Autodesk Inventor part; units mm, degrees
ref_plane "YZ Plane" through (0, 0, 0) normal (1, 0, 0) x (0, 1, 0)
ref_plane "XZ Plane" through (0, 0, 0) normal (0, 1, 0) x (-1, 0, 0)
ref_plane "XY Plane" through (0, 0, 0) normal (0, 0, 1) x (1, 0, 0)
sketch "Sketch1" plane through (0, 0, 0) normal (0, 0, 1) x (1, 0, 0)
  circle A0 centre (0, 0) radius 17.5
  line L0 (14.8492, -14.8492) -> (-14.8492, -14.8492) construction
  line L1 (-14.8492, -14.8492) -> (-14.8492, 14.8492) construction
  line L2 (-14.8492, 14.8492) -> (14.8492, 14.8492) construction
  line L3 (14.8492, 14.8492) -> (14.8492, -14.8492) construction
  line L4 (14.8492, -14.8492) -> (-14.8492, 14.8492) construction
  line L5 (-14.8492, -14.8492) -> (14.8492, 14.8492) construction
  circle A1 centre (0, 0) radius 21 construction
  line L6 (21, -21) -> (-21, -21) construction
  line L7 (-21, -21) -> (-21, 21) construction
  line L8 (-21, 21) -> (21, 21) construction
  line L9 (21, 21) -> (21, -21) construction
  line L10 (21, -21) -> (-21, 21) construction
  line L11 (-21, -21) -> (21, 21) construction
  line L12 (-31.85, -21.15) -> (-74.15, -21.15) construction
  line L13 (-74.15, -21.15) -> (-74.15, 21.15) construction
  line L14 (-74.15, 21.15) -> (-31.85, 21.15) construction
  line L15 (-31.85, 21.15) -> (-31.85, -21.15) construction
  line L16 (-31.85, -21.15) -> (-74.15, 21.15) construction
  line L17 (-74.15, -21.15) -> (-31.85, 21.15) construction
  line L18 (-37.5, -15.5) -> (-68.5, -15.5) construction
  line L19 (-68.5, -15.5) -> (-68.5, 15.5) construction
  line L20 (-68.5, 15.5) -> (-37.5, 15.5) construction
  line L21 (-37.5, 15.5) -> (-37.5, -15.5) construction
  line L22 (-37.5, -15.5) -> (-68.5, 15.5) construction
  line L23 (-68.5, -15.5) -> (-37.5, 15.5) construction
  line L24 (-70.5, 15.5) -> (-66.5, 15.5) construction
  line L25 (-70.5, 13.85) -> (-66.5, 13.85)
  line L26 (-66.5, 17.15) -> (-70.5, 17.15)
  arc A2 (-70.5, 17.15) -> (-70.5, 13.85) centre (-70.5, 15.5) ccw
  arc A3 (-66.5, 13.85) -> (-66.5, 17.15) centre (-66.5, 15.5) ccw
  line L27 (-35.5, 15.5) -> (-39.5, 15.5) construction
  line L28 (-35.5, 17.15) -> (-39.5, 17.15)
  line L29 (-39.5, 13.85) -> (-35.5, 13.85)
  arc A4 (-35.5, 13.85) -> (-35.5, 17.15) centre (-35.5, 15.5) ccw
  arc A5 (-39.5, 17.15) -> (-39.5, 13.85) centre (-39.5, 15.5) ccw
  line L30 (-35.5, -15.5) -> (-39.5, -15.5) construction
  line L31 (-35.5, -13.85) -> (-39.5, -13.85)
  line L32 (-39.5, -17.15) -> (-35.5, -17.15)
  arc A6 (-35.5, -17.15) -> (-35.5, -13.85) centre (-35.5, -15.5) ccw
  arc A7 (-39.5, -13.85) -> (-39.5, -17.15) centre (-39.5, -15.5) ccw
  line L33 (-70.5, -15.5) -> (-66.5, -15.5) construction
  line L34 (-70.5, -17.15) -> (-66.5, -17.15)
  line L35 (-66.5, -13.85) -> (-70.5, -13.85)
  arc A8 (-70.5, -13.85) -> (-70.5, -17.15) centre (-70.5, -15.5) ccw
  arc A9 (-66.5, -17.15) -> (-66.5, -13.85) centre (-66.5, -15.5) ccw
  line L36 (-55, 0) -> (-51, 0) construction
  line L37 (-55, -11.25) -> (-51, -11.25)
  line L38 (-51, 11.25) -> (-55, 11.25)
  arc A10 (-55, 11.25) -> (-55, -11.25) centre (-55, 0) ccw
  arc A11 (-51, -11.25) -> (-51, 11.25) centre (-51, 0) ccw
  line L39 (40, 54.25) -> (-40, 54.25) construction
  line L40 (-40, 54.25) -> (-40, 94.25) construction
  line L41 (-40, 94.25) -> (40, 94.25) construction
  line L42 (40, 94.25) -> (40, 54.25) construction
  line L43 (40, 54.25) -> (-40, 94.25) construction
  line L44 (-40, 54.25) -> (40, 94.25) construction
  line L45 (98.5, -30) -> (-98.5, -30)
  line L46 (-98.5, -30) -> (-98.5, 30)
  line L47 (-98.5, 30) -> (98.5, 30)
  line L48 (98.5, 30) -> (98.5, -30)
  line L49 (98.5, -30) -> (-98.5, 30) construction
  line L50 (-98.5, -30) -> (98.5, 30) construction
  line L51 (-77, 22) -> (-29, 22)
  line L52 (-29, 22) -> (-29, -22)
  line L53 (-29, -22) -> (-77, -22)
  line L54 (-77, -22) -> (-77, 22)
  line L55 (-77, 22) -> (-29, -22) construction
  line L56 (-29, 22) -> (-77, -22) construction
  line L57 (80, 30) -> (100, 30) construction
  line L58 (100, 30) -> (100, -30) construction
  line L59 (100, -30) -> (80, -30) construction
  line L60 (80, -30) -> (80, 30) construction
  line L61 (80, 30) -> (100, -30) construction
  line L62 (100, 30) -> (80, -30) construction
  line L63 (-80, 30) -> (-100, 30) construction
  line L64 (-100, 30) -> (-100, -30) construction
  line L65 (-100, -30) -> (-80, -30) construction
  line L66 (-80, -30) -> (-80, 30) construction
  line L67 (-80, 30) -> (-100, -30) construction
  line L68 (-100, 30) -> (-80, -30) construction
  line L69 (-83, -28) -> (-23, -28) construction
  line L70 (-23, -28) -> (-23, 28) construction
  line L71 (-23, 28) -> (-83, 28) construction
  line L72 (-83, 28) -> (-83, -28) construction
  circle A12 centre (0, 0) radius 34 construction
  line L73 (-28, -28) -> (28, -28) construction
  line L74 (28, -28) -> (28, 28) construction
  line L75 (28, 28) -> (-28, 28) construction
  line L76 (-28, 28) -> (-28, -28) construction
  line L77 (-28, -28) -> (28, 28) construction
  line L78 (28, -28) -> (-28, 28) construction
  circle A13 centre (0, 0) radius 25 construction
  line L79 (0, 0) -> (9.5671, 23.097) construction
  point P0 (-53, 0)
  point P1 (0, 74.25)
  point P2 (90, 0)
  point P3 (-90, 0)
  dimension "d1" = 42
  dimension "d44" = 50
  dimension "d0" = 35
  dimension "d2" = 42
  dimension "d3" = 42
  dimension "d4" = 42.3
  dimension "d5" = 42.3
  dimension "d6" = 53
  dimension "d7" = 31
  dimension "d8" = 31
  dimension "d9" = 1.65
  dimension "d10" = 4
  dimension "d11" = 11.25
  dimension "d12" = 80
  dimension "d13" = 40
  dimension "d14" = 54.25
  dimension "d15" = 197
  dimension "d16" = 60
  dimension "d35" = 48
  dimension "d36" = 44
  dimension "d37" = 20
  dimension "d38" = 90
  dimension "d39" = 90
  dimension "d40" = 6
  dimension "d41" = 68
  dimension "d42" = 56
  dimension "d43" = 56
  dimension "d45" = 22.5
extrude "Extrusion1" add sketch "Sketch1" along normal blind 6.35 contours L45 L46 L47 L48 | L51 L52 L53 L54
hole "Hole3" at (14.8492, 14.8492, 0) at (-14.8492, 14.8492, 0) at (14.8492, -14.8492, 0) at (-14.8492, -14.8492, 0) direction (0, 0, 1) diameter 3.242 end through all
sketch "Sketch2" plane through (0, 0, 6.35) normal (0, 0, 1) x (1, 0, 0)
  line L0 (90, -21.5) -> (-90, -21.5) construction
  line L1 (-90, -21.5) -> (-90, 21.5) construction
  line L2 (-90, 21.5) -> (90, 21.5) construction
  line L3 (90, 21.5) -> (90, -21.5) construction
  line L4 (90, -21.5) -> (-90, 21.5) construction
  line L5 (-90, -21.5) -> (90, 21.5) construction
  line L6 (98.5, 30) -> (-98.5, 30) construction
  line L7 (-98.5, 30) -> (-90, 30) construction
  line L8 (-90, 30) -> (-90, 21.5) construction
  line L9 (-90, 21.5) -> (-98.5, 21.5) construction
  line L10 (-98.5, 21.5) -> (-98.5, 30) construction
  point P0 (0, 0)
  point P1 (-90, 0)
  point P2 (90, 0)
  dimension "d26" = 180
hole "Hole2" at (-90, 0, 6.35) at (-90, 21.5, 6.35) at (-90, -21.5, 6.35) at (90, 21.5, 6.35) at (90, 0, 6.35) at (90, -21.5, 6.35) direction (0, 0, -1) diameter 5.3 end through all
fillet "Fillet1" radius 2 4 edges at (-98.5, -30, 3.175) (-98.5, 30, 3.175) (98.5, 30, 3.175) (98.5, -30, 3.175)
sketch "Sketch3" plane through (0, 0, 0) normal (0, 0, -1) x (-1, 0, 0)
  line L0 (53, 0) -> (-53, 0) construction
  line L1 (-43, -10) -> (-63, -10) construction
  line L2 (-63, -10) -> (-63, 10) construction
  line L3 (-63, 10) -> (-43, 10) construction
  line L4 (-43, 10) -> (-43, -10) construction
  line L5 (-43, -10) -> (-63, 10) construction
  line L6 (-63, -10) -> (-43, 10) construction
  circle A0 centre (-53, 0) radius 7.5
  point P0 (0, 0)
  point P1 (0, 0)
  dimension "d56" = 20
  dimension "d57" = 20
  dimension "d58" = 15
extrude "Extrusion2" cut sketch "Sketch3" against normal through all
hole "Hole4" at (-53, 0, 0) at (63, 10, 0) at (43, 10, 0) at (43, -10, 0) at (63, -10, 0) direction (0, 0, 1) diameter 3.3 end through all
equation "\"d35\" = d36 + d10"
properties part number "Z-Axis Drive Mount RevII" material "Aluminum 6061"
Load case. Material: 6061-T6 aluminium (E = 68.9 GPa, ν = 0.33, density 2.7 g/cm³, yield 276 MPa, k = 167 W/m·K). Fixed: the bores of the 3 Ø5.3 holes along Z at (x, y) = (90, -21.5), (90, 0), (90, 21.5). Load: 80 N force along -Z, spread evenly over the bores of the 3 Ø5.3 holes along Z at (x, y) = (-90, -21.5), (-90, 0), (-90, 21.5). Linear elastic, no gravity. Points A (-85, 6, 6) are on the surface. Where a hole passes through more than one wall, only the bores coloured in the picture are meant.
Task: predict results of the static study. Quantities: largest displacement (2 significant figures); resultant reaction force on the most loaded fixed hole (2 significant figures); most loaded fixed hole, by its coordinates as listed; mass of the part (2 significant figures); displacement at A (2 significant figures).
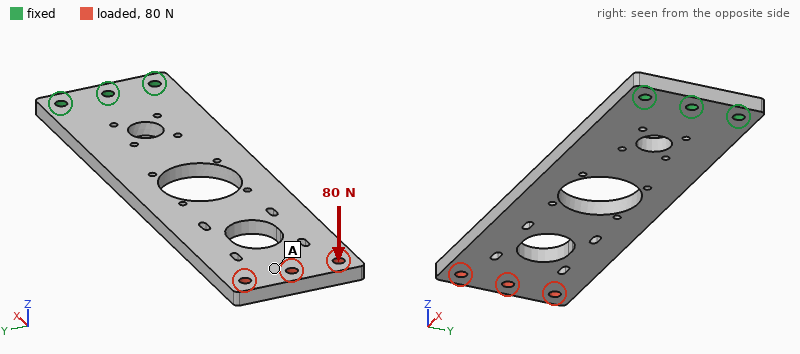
2.4 mm
150 N
(90, 0)
170 g
2.2 mm
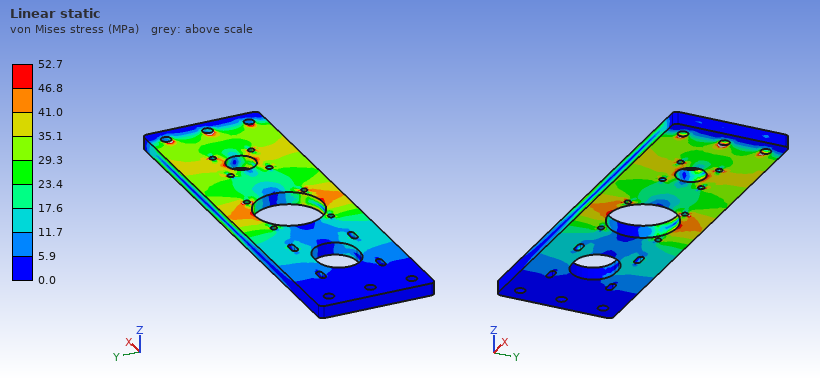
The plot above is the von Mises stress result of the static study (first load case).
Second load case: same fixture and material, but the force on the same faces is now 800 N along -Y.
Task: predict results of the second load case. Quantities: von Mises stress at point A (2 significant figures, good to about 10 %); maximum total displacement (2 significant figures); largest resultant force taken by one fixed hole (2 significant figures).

5.2 MPa
0.28 mm
3.2 kN
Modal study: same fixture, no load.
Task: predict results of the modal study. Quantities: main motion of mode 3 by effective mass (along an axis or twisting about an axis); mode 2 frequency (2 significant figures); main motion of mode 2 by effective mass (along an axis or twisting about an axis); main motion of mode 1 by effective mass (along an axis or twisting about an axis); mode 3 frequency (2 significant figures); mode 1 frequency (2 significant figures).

along Z
810 Hz
twisting about X
along Z
860 Hz
140 Hz
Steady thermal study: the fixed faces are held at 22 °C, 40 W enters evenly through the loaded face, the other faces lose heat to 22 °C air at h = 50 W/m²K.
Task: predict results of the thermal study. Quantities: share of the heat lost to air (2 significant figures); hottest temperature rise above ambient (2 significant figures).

78 %
65 K
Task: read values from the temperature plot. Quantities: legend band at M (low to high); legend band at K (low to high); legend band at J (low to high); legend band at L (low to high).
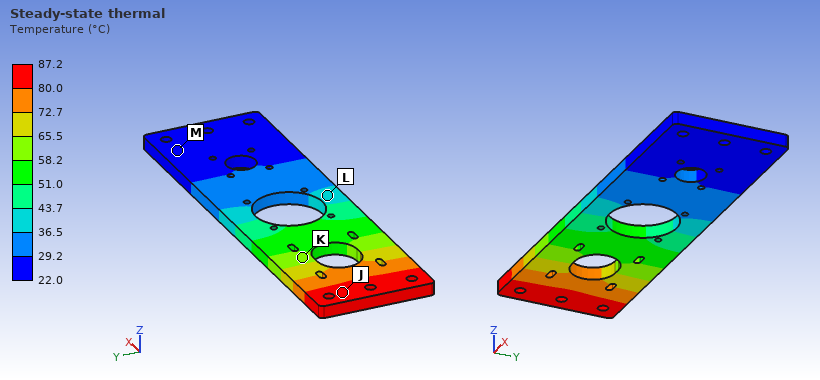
22.0 to 29.2 °C
58.2 to 65.5 °C
80.0 to 87.2 °C
36.5 to 43.7 °C
